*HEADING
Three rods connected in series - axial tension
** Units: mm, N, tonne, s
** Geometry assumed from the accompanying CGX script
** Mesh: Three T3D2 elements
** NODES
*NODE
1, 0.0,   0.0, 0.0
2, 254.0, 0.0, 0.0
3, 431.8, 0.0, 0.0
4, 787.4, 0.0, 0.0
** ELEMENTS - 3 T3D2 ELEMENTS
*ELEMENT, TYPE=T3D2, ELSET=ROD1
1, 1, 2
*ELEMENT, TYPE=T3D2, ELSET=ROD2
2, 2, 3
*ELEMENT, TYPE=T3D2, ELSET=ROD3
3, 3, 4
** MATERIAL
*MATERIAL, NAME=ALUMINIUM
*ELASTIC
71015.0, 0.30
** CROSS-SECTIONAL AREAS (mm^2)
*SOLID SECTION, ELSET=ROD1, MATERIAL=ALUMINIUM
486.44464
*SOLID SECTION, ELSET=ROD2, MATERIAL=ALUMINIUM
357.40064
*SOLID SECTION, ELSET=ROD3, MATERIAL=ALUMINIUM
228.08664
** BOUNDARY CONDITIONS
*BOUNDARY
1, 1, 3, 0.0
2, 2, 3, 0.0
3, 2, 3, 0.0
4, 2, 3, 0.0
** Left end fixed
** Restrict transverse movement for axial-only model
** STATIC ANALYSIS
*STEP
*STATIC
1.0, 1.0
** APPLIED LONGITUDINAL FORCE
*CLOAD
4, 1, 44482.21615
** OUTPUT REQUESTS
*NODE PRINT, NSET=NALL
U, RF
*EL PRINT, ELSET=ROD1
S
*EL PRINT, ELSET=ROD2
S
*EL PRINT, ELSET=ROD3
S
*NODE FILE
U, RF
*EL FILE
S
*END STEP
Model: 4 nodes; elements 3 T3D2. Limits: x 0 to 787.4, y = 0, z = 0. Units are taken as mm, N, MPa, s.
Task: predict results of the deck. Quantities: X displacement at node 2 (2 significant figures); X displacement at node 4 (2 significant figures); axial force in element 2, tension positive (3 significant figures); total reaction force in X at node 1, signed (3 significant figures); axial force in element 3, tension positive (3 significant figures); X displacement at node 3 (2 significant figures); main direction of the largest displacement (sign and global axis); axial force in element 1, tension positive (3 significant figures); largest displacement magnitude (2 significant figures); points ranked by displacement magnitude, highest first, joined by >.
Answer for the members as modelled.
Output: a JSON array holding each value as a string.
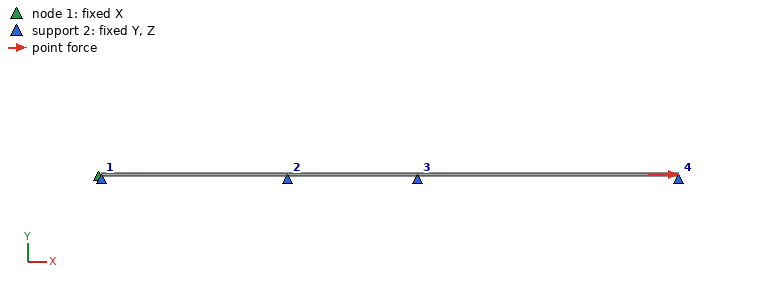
["0.33 mm", "1.6 mm", "44500 N", "-44500 N", "44500 N", "0.64 mm", "+X", "44500 N", "1.6 mm", "node 4 > node 3 > node 2 > node 1"]
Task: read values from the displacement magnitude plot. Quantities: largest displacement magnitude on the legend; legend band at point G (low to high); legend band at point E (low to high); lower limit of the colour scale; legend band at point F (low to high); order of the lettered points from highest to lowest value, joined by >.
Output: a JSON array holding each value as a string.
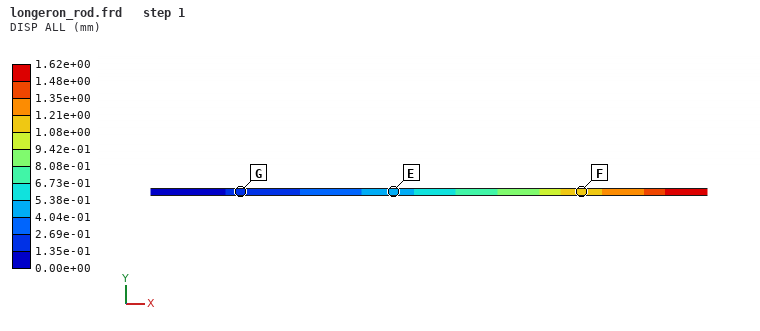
["1.62e+00 mm", "1.35e-01 to 2.69e-01 mm", "4.04e-01 to 5.38e-01 mm", "0.00e+00 mm", "1.08e+00 to 1.21e+00 mm", "F > E > G"]
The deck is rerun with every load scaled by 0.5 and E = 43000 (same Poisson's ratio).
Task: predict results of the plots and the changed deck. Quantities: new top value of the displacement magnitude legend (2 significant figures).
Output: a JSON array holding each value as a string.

["1.3 mm"]
